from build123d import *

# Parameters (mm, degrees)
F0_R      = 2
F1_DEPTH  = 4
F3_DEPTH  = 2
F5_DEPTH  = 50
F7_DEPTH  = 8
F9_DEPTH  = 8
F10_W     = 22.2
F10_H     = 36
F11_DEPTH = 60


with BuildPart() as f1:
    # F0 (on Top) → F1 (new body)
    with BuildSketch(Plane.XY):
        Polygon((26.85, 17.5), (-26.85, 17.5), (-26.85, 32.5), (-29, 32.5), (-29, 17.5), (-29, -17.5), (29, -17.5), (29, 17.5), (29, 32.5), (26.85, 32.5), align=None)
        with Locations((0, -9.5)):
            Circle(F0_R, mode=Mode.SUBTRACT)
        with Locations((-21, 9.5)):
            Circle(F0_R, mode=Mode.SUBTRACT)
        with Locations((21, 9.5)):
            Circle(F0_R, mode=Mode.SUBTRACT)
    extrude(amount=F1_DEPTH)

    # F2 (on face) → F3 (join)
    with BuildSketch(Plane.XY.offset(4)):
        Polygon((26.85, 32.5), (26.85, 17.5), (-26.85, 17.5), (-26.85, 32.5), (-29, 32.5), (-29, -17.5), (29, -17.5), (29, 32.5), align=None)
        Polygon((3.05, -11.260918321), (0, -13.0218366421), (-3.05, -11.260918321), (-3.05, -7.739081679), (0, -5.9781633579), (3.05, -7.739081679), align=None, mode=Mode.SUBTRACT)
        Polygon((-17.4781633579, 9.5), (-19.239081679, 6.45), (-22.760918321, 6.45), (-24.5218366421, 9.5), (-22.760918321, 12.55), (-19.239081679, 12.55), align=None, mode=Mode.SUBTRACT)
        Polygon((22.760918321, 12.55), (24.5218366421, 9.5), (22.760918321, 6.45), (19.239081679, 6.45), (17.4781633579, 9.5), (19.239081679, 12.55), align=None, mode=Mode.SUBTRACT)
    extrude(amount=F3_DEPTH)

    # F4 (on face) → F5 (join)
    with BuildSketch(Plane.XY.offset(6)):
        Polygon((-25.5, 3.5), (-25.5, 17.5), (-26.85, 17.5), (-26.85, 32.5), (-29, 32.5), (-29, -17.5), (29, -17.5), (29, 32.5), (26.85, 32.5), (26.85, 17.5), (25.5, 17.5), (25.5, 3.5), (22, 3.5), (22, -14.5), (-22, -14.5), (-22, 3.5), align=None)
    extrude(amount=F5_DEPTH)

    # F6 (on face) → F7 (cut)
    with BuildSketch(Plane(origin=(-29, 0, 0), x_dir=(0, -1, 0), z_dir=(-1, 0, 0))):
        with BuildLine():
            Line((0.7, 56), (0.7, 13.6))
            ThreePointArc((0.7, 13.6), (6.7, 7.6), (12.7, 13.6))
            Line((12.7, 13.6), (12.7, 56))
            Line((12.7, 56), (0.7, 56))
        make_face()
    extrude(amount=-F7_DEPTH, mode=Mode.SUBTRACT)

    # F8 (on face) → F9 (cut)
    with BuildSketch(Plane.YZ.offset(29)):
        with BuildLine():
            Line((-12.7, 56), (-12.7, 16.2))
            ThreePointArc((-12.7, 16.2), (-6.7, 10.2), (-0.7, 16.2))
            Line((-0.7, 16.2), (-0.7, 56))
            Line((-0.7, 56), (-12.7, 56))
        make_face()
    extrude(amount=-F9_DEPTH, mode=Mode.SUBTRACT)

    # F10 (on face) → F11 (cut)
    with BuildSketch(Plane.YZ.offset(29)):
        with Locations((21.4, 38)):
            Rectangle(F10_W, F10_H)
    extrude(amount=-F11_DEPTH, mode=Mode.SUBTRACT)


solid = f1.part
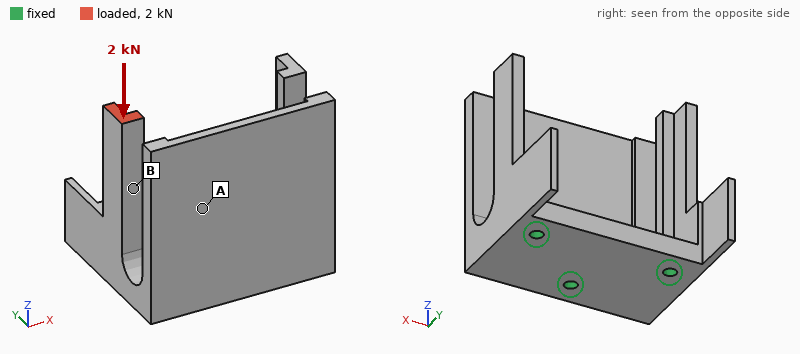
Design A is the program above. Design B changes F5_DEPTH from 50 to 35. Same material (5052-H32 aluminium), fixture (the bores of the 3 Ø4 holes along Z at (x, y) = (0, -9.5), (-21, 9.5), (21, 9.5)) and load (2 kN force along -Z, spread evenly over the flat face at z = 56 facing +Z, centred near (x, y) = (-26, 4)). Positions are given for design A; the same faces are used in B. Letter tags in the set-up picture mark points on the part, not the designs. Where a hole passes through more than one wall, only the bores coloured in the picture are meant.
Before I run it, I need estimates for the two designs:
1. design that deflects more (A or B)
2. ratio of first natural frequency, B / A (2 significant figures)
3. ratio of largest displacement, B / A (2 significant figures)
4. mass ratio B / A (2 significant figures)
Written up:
A
2.0
0.74
0.85
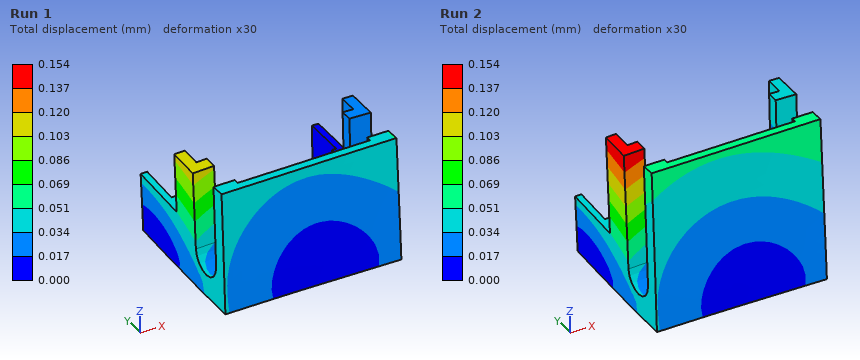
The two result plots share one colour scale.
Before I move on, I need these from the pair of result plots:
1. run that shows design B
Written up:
Run 1
